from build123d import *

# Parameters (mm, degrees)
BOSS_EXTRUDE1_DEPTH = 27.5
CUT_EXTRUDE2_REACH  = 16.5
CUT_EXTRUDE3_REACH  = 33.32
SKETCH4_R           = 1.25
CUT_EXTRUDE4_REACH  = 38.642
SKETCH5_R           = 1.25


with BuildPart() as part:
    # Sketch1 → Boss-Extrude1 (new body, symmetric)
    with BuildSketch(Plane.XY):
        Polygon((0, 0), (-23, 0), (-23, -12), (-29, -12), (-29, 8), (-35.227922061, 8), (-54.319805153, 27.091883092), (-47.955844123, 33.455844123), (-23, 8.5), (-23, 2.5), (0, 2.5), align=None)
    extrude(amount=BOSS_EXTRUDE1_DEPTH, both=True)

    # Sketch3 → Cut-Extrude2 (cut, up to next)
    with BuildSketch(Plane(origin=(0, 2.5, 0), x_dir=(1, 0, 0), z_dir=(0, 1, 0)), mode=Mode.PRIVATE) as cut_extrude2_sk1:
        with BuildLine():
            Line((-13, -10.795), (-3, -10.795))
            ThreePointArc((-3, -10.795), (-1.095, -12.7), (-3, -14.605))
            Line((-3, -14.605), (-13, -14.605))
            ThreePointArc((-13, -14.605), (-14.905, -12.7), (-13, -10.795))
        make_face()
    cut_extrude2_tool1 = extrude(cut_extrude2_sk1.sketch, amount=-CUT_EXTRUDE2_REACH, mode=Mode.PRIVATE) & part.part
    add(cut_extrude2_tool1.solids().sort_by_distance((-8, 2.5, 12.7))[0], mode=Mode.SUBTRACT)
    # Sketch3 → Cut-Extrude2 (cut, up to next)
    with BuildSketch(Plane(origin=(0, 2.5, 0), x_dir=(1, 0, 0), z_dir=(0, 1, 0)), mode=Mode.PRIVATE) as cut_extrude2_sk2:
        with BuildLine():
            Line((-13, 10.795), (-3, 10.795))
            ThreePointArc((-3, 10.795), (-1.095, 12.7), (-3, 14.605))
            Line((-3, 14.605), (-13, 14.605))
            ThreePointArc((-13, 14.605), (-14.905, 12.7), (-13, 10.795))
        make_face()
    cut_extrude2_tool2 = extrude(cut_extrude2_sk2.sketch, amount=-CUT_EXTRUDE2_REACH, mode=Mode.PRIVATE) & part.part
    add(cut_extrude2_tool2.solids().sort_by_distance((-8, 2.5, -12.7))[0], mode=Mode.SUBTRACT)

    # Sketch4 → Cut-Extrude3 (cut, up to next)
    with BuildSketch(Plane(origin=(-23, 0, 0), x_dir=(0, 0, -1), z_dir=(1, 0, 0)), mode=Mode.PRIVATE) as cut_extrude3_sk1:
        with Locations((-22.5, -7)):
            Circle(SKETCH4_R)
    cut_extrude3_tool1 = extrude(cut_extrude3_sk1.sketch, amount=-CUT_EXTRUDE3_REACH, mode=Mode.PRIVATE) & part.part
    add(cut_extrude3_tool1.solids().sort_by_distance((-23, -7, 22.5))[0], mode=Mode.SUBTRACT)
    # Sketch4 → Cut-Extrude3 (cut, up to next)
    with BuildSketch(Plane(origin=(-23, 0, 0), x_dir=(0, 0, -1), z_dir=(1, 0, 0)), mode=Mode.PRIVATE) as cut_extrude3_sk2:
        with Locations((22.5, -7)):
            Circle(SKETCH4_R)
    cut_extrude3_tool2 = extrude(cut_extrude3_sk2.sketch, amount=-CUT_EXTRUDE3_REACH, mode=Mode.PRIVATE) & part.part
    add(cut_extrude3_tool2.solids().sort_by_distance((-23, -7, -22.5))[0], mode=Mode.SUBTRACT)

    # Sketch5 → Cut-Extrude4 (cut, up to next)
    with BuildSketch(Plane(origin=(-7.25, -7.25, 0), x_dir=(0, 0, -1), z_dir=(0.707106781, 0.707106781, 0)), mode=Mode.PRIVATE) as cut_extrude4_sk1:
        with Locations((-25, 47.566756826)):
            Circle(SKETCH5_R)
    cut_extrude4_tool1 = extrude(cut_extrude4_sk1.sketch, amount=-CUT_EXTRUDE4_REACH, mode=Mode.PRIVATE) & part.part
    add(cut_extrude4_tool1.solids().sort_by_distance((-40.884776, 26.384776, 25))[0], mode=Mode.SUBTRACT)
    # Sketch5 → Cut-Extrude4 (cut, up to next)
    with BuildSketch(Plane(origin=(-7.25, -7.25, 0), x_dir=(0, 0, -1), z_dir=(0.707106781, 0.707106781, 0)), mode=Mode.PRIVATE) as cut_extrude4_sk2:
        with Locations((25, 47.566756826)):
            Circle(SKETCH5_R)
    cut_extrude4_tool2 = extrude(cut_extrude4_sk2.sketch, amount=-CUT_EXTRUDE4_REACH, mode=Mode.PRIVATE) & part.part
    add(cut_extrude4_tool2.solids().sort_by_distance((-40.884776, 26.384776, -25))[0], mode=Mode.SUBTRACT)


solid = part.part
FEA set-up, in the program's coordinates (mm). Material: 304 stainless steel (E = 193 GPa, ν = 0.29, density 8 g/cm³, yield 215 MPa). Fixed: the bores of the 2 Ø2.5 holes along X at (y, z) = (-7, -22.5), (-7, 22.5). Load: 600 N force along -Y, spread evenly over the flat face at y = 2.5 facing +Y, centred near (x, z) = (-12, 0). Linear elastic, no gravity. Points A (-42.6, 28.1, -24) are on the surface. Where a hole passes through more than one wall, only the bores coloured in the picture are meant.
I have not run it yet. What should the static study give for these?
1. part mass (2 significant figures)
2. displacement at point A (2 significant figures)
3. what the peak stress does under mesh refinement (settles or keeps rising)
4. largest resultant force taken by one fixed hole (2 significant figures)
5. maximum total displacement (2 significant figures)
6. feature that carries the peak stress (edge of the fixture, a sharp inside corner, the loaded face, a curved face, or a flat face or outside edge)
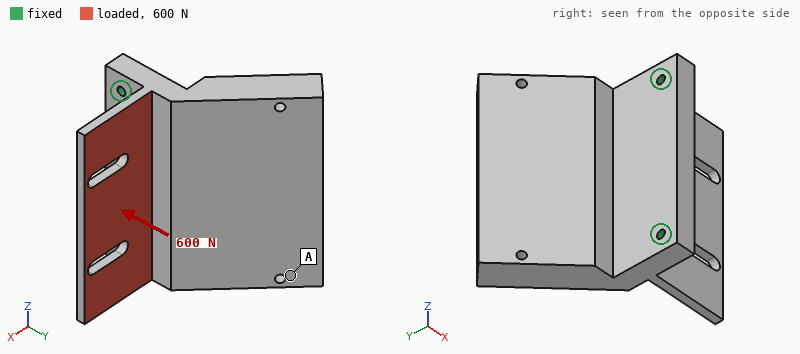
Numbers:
200 g
26 µm
keeps rising
310 N
90 µm
edge of the fixture
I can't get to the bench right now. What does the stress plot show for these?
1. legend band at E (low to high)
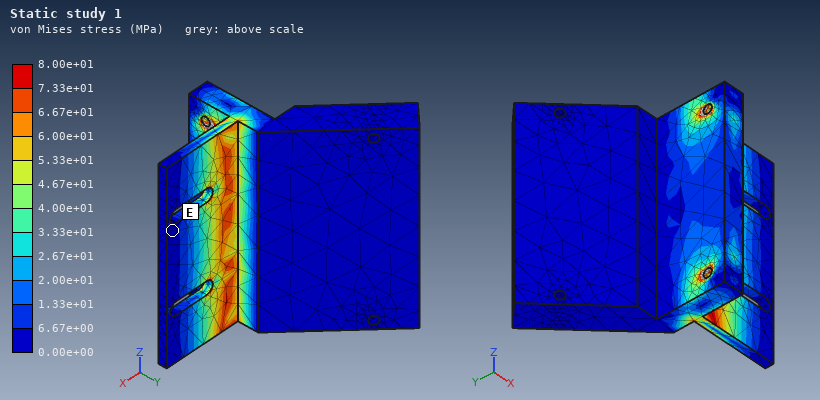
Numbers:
0.00e+00 to 6.67e+00 MPa
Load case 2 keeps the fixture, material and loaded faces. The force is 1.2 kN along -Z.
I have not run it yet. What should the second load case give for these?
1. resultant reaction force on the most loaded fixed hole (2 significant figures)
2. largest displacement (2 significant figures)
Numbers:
740 N
11 µm
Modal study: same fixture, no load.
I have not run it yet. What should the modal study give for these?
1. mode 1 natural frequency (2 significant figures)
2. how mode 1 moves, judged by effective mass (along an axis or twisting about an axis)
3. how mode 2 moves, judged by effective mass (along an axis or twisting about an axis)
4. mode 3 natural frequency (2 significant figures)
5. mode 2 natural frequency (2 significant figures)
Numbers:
1400 Hz
along X
along Y
4100 Hz
3600 Hz
